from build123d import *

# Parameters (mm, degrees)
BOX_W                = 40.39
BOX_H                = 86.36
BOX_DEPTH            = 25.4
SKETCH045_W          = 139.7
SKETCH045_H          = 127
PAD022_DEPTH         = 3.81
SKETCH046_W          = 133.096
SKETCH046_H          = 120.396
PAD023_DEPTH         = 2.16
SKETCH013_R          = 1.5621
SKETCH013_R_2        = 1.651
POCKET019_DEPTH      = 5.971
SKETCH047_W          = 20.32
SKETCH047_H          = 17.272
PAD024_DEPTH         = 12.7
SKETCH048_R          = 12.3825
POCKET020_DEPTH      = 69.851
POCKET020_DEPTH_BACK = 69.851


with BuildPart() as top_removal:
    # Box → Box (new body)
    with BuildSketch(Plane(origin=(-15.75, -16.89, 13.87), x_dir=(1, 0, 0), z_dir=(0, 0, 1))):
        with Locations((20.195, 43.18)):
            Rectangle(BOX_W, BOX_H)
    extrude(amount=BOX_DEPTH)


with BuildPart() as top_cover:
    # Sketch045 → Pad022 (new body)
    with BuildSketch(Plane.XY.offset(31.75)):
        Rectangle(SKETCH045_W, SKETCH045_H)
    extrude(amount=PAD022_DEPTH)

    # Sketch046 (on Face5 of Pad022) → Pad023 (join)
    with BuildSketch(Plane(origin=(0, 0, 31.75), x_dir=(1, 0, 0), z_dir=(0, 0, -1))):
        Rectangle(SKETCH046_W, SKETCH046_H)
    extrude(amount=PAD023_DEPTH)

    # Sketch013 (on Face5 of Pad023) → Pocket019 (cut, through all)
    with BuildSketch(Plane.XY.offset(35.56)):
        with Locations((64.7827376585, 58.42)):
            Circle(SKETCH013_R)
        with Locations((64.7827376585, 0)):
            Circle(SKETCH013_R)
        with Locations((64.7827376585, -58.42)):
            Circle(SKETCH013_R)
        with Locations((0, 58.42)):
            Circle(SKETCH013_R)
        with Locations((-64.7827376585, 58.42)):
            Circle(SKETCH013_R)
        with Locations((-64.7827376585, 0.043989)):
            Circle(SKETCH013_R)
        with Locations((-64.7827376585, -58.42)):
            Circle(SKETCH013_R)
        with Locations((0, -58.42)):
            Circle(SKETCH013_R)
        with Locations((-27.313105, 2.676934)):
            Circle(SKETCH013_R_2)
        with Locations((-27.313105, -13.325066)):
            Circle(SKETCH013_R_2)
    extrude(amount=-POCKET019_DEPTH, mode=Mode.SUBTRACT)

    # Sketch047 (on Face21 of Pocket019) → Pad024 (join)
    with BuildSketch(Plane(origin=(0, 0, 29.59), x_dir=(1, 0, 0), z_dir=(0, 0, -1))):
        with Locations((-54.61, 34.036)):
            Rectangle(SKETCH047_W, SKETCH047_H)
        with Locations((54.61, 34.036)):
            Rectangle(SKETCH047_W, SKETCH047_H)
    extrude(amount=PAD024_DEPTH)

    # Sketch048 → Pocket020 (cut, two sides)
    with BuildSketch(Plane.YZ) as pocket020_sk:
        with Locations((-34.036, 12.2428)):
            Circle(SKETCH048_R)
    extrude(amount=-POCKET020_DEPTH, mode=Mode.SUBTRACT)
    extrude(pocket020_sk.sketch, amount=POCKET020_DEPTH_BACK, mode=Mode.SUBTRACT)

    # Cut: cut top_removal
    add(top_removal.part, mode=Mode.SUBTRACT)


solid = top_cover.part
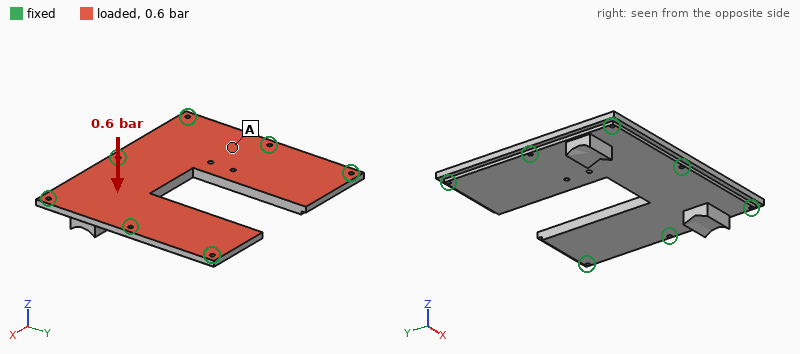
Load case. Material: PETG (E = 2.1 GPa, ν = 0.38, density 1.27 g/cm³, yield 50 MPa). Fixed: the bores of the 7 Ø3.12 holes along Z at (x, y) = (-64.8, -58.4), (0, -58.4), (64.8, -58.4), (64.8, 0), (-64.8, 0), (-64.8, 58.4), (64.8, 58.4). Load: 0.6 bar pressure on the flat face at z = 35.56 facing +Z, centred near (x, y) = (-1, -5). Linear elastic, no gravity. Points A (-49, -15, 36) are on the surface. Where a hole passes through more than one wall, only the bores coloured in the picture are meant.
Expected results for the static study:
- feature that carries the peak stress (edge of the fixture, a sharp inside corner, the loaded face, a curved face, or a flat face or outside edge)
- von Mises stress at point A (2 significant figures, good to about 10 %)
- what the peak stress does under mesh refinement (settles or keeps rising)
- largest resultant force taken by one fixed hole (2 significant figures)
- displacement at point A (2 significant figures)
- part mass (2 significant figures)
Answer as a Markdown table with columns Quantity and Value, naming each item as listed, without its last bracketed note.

| Quantity | Value |
|---|---|
| feature that carries the peak stress | edge of the fixture |
| von Mises stress at point A | 4.9 MPa |
| what the peak stress does under mesh refinement | keeps rising |
| largest resultant force taken by one fixed hole | 220 N |
| displacement at point A | 0.32 mm |
| part mass | 110 g |
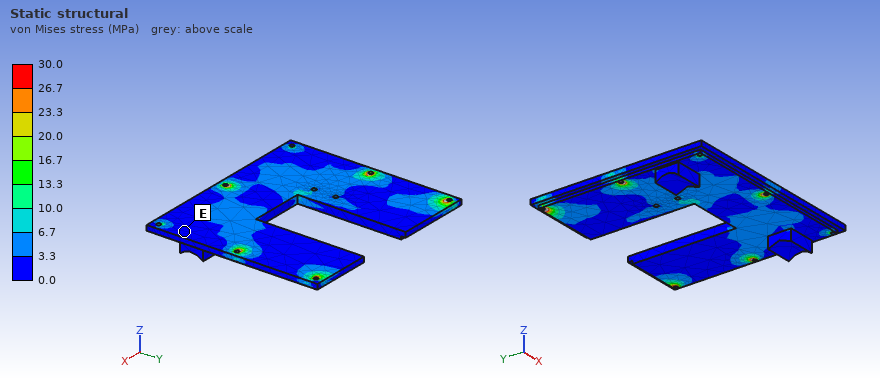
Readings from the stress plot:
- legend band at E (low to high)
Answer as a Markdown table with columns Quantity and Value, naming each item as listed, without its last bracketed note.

| Quantity | Value |
|---|---|
| legend band at E | 0.0 to 3.3 MPa |
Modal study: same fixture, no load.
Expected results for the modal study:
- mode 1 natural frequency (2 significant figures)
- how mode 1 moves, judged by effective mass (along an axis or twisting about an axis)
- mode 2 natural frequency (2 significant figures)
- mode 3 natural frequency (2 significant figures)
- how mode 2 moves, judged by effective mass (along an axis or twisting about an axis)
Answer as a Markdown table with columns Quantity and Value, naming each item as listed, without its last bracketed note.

| Quantity | Value |
|---|---|
| mode 1 natural frequency | 450 Hz |
| how mode 1 moves, judged by effective mass | along Z |
| mode 2 natural frequency | 590 Hz |
| mode 3 natural frequency | 860 Hz |
| how mode 2 moves, judged by effective mass | along Z |
